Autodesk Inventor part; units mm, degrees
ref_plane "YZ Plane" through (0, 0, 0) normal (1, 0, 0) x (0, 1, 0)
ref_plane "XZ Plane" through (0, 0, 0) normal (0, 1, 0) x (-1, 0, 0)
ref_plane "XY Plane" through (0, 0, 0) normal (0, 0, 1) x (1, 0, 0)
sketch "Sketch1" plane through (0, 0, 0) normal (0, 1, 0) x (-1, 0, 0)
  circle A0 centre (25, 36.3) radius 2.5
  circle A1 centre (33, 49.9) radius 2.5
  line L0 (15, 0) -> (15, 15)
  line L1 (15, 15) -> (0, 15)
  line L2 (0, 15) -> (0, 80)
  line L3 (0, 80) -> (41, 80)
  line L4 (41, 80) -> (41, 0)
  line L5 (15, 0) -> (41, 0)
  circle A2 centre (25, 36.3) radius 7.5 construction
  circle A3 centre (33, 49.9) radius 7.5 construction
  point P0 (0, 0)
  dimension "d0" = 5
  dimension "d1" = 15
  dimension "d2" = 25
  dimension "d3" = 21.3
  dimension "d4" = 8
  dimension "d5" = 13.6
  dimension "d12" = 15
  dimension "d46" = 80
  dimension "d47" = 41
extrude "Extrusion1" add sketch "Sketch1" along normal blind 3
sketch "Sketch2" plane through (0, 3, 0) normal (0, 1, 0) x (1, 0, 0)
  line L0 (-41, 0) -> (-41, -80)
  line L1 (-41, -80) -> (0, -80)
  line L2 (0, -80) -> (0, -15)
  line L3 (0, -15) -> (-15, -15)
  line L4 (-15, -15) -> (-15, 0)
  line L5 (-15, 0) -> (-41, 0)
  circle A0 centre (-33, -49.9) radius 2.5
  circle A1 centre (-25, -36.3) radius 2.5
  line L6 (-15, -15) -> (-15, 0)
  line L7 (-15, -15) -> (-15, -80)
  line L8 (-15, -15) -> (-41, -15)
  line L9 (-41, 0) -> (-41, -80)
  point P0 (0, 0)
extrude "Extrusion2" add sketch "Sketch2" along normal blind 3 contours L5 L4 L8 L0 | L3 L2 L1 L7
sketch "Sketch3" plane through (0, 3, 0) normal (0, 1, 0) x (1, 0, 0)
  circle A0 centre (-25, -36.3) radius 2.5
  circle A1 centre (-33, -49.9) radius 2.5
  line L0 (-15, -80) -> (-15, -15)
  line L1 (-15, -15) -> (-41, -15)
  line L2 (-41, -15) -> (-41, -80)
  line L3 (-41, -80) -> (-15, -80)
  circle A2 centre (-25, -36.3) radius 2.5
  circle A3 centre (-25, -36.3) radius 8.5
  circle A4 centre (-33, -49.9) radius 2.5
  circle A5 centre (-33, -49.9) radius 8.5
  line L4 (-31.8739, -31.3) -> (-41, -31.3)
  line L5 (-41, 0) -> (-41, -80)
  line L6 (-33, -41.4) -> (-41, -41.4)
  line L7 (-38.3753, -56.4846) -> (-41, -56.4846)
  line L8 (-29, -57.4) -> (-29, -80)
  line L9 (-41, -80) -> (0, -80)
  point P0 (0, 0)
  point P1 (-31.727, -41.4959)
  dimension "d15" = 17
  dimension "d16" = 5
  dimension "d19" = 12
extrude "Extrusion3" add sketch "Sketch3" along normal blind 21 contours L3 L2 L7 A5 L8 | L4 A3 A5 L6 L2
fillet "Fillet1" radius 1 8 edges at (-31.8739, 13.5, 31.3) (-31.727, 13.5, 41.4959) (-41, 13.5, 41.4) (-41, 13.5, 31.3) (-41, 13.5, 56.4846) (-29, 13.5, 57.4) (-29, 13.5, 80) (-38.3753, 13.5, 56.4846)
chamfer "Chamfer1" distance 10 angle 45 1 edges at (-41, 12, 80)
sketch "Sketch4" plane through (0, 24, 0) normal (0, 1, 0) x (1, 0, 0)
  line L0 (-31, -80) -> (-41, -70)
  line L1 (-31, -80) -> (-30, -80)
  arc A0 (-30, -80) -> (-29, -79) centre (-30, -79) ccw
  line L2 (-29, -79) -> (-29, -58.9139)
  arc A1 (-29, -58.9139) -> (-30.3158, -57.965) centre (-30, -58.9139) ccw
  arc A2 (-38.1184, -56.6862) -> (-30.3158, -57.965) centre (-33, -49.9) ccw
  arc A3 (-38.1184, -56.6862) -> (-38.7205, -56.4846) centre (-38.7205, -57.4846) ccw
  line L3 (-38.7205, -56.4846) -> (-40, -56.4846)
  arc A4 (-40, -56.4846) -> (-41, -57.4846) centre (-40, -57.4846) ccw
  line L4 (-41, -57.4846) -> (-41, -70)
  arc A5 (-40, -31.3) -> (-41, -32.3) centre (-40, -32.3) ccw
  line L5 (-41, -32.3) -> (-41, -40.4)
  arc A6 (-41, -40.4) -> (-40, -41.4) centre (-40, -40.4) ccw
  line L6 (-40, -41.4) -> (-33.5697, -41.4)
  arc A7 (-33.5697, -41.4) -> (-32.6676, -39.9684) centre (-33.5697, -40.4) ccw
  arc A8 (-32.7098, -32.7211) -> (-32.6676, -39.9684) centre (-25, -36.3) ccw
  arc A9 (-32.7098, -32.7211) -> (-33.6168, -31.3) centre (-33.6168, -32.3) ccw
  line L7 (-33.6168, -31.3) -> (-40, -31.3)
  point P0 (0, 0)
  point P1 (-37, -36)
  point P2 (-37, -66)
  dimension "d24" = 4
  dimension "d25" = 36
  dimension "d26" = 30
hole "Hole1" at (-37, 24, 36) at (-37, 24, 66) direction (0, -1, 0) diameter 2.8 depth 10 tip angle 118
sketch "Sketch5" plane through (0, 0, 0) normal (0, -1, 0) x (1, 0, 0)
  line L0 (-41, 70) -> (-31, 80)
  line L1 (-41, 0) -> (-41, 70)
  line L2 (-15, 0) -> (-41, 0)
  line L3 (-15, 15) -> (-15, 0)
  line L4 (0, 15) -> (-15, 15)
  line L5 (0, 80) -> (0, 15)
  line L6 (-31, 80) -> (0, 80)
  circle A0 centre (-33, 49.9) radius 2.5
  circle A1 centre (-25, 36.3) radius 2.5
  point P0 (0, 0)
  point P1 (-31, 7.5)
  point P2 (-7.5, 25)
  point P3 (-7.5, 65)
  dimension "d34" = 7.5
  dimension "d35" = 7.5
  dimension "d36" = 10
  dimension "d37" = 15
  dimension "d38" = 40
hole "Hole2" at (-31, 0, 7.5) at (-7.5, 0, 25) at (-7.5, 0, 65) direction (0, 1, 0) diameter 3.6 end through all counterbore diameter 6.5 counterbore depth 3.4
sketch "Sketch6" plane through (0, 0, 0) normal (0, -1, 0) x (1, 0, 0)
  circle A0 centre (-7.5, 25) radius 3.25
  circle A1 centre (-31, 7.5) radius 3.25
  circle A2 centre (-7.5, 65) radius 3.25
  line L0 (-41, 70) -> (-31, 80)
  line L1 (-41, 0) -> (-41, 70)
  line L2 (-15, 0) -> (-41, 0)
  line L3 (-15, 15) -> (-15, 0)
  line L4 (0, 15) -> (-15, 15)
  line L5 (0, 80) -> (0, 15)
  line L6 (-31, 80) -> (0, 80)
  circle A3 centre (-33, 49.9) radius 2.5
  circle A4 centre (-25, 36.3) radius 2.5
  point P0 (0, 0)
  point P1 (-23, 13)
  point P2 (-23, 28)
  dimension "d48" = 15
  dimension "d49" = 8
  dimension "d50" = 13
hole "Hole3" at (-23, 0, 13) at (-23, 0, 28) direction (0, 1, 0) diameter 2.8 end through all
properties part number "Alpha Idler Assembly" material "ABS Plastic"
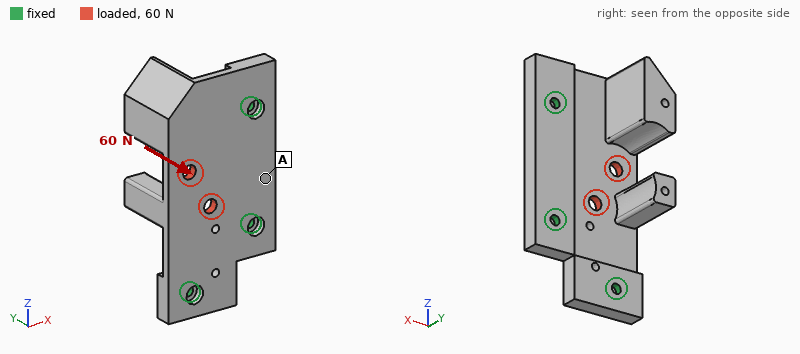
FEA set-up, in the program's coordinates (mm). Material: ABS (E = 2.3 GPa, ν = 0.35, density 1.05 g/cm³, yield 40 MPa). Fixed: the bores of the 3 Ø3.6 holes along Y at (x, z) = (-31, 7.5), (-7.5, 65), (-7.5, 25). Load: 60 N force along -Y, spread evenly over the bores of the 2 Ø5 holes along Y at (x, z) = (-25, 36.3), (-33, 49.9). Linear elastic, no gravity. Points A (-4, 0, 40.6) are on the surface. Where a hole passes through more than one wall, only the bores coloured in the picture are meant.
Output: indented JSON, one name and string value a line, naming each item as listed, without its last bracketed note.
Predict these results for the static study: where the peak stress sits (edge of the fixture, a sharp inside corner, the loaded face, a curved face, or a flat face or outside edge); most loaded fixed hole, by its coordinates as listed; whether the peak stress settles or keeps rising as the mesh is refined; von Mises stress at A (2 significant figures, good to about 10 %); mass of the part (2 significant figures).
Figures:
{
  "where the peak stress sits": "edge of the fixture",
  "most loaded fixed hole, by its coordinates as listed": "(-7.5, 65)",
  "whether the peak stress settles or keeps rising as the mesh is refined": "keeps rising",
  "von Mises stress at A": "1.9 MPa",
  "mass of the part": "20 g"
}
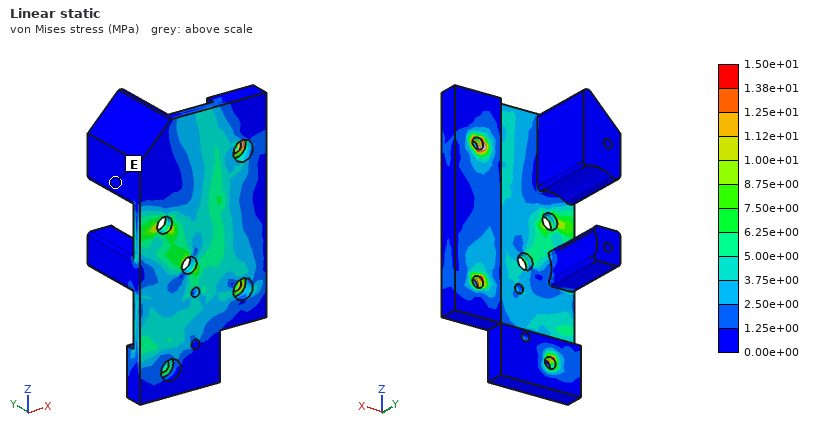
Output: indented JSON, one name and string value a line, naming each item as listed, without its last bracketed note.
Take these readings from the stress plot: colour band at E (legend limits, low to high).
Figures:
{
  "colour band at E": "0.00e+00 to 1.25e+00 MPa"
}
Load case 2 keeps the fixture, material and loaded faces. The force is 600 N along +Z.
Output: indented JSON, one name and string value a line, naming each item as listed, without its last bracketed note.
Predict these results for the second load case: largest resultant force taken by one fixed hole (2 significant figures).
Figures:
{
  "largest resultant force taken by one fixed hole": "260 N"
}
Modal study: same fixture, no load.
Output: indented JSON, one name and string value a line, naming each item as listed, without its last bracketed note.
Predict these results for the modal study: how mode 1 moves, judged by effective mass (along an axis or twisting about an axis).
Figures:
{
  "how mode 1 moves, judged by effective mass": "along Y"
}
